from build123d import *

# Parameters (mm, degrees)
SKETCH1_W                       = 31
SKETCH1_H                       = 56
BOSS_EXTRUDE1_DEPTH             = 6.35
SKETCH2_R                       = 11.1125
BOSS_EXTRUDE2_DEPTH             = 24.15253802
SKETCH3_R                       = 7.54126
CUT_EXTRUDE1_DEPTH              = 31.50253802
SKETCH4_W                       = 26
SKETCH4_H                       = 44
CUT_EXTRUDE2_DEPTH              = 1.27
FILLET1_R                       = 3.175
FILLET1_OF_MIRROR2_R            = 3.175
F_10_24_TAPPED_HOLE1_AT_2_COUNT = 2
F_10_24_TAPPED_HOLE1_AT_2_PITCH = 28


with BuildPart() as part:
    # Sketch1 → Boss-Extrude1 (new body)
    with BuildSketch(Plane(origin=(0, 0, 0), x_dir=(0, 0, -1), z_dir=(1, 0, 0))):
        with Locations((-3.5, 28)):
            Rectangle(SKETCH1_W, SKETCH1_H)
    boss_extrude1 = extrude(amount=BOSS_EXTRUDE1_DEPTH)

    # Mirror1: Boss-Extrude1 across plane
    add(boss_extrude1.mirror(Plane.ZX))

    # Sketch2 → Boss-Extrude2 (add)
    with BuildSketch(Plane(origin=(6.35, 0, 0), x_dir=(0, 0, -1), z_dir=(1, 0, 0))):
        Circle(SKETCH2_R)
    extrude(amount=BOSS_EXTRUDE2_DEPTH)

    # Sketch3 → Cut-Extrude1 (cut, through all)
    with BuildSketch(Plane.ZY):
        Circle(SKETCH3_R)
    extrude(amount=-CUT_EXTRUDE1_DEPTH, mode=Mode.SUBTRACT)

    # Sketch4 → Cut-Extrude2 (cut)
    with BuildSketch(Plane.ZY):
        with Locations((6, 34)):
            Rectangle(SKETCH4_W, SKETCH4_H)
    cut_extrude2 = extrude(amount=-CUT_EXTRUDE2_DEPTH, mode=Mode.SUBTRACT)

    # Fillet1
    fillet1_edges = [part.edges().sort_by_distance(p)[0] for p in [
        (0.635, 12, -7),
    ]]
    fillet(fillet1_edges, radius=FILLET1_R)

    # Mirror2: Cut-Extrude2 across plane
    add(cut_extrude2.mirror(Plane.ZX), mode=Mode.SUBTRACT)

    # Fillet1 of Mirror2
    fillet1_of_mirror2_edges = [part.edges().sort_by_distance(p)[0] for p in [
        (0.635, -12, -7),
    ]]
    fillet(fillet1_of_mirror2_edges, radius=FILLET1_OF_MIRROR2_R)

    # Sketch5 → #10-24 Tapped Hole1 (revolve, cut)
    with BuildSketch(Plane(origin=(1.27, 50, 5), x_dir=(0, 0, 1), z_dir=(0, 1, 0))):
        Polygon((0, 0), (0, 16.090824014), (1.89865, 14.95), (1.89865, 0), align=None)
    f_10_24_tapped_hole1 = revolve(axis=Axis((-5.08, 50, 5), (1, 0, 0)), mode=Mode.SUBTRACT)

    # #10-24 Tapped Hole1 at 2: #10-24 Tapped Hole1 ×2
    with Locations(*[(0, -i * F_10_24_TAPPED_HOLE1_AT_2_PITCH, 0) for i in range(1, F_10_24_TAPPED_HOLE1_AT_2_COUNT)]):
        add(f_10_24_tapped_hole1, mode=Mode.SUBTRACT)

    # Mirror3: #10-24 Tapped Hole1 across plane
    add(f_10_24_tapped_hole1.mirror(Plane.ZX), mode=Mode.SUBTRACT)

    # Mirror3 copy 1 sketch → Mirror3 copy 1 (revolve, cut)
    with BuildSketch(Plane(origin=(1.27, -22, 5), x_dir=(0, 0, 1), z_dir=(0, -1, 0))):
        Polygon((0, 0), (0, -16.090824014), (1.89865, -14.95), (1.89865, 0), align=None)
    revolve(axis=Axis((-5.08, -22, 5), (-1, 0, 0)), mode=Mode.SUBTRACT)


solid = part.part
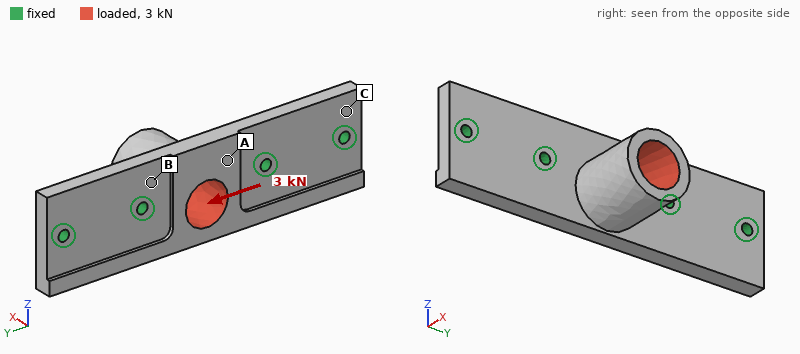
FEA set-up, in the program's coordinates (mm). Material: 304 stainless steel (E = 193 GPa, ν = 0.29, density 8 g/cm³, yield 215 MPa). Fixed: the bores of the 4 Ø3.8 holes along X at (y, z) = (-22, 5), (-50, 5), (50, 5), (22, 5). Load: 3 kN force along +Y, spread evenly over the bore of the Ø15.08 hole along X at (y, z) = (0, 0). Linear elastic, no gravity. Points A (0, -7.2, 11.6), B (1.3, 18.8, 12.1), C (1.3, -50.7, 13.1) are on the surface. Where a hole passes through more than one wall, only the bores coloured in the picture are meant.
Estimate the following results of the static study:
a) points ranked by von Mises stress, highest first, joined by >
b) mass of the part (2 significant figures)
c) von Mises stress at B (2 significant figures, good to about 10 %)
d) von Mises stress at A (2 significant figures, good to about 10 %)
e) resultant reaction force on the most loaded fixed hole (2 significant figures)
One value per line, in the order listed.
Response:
A > B > C
180 g
12 MPa
22 MPa
1.6 kN
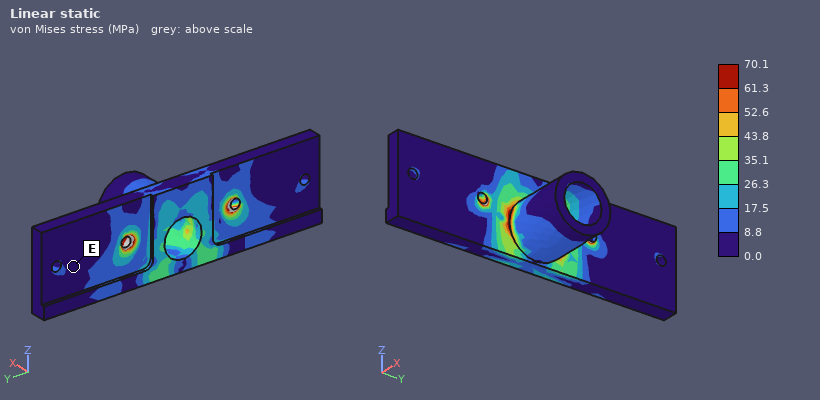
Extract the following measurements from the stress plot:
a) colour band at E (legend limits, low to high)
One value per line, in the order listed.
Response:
0.0 to 8.8 MPa
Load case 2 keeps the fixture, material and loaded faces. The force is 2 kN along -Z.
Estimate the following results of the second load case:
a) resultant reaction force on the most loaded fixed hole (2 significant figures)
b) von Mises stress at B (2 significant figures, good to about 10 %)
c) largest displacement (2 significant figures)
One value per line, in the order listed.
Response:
1.1 kN
25 MPa
58 µm
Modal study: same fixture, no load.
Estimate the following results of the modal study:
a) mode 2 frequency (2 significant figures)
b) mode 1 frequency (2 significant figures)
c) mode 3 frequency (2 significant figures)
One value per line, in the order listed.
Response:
9000 Hz
4400 Hz
9300 Hz
